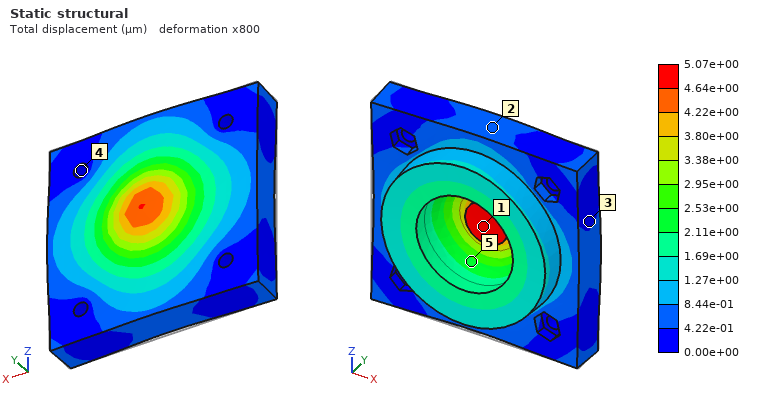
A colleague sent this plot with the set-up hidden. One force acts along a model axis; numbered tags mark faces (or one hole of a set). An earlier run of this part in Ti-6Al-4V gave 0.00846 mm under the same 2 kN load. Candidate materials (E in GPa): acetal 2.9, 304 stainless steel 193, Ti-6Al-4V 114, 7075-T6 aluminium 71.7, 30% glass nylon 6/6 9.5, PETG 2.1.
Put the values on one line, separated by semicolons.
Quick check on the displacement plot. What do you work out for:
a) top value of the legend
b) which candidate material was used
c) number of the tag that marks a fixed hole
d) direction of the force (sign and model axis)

5.07e+00 µm; 304 stainless steel; 4; +Y
